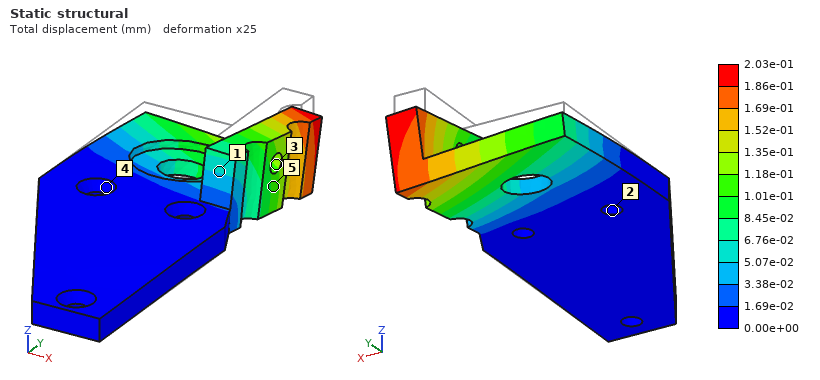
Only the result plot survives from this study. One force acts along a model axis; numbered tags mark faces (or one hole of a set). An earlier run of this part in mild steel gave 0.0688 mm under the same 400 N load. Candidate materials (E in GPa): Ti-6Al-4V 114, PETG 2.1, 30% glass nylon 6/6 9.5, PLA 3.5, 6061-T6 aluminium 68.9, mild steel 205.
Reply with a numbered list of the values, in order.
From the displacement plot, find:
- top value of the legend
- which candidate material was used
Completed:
1. 2.03e-01 mm
2. 6061-T6 aluminium
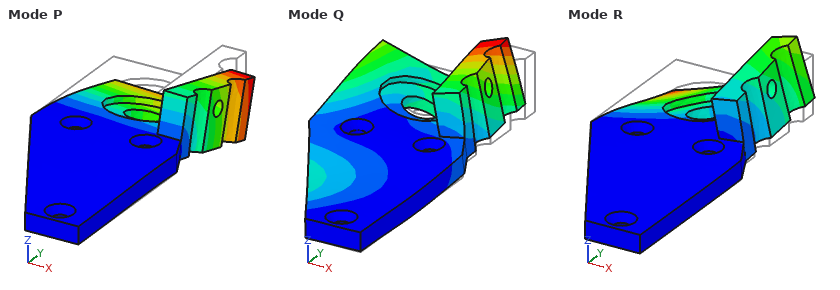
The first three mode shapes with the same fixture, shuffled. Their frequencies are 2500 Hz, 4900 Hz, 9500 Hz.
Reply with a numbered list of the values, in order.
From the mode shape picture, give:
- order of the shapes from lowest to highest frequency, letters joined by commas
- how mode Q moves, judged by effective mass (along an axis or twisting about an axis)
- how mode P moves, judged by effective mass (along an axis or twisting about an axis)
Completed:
1. P, R, Q
2. along X
3. along Z
